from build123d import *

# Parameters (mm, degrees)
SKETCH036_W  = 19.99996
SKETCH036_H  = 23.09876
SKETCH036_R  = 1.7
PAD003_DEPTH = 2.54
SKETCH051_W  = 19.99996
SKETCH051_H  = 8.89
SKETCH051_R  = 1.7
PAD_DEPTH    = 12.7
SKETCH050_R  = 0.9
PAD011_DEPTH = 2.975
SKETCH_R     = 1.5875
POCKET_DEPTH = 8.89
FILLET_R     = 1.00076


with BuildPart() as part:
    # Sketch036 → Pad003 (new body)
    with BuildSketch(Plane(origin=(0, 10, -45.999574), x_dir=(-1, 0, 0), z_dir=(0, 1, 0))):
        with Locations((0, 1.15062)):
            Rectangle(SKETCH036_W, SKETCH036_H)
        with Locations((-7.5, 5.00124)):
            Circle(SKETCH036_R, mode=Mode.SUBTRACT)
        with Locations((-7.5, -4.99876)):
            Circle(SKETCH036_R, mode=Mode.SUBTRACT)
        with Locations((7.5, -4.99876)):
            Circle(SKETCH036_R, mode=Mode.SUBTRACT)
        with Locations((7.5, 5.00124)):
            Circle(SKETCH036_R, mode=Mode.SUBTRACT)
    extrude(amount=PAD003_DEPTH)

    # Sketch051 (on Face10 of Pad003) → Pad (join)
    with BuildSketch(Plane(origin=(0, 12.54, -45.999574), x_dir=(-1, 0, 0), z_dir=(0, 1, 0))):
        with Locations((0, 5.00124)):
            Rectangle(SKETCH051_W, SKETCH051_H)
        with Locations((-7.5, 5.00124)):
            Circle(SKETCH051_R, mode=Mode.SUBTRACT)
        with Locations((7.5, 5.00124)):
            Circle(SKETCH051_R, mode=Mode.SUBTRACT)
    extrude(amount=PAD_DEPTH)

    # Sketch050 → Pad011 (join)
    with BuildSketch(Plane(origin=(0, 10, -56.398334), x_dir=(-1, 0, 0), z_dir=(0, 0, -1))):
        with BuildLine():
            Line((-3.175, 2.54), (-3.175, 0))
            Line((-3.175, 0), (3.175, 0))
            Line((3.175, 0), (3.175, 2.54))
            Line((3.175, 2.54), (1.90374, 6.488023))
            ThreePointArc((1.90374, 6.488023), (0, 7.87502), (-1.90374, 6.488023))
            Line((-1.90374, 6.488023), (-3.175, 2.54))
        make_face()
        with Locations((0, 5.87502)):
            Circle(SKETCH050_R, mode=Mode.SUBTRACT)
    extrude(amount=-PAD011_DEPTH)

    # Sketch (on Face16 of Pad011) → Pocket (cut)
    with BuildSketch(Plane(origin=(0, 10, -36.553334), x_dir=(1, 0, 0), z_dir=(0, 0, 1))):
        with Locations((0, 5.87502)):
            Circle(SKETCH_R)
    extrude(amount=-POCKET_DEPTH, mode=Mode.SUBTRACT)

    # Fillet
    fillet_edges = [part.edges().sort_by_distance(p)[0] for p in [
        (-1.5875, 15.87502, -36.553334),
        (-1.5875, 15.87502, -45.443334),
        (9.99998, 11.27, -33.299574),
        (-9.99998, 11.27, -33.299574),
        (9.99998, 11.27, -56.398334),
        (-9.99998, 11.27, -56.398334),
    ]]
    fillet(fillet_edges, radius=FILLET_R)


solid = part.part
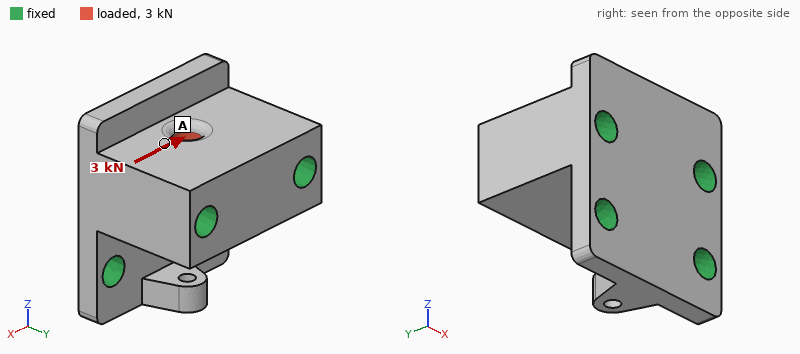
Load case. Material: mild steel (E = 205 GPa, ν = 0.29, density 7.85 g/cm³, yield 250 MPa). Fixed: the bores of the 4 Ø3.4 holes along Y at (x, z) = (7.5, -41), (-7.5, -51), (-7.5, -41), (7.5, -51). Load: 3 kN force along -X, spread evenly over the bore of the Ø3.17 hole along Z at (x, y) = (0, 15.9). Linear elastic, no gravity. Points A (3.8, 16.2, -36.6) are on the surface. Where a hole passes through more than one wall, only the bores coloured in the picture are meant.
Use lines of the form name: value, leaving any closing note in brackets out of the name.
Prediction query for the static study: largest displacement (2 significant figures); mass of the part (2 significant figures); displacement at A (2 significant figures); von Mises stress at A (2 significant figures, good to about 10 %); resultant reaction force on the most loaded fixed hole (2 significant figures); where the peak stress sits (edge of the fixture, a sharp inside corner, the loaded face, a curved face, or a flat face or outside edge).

largest displacement: 0.85 µm
mass of the part: 24 g
displacement at A: 0.39 µm
von Mises stress at A: 12 MPa
resultant reaction force on the most loaded fixed hole: 1.5 kN
where the peak stress sits: the loaded face
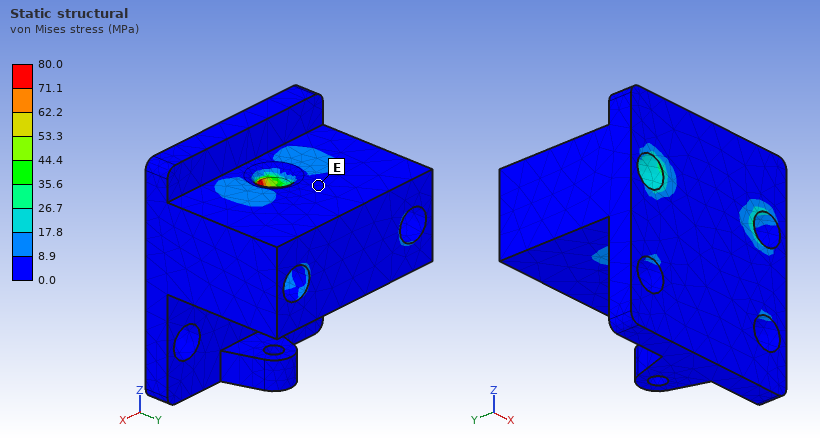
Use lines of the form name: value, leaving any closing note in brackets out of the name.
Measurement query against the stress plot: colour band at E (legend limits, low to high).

colour band at E: 0.0 to 8.9 MPa
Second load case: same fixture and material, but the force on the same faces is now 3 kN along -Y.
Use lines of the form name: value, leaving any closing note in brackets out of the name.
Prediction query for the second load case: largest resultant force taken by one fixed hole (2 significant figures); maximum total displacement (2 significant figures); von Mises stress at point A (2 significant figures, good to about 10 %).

largest resultant force taken by one fixed hole: 1.5 kN
maximum total displacement: 1.4 µm
von Mises stress at point A: 18 MPa
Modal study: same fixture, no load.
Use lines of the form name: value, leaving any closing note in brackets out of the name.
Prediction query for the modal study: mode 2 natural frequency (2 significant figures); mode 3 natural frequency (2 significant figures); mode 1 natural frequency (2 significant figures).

mode 2 natural frequency: 63 kHz
mode 3 natural frequency: 70 kHz
mode 1 natural frequency: 38 kHz
